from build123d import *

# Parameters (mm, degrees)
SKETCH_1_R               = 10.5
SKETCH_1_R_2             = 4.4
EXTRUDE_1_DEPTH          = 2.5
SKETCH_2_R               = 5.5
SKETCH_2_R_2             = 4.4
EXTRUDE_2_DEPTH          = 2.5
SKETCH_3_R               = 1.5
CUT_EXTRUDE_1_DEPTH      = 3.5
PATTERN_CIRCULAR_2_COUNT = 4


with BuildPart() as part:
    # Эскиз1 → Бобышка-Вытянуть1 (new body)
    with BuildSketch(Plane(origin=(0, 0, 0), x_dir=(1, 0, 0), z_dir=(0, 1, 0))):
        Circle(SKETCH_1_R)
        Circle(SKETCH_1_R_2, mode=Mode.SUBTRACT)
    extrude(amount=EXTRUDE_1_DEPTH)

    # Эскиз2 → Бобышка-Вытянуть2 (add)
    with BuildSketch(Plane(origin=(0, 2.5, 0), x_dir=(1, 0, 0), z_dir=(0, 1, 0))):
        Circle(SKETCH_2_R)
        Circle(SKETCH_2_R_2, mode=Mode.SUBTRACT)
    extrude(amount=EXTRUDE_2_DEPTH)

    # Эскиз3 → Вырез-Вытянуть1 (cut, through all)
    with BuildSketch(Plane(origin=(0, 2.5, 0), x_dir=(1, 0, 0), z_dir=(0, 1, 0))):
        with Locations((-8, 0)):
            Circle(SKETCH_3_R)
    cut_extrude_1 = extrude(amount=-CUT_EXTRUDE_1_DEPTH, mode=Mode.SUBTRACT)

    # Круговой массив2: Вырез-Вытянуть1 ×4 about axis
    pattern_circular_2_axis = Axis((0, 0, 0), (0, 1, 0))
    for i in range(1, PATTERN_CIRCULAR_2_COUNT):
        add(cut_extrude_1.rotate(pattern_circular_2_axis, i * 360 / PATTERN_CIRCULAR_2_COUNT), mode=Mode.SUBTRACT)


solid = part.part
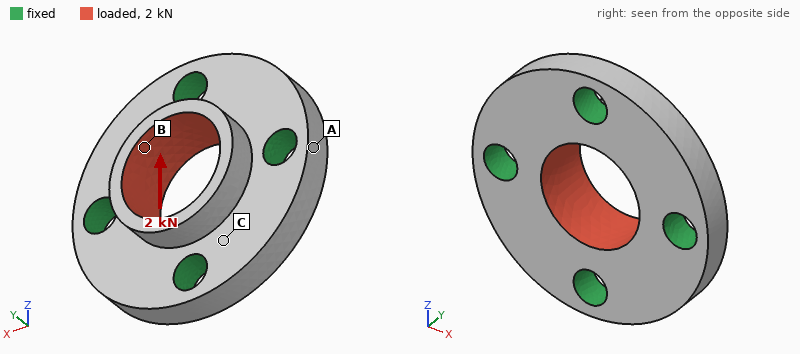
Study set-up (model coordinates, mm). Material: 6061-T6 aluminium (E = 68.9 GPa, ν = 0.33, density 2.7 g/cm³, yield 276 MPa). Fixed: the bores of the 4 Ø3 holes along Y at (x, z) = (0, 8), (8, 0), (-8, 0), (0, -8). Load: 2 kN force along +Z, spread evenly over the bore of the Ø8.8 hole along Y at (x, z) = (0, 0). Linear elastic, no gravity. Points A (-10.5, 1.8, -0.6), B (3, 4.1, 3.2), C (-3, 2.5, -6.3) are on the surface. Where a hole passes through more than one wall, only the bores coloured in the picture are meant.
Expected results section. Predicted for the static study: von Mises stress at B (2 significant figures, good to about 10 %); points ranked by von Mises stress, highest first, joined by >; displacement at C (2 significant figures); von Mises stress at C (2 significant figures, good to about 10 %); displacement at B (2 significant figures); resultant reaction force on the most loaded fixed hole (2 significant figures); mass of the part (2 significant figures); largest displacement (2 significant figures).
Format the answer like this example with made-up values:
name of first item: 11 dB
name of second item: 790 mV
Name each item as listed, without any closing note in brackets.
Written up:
von Mises stress at B: 47 MPa
points ranked by von Mises stress, highest first, joined by >: B > C > A
displacement at C: 1.5 µm
von Mises stress at C: 29 MPa
displacement at B: 6.8 µm
resultant reaction force on the most loaded fixed hole: 550 N
mass of the part: 2.0 g
largest displacement: 9.0 µm
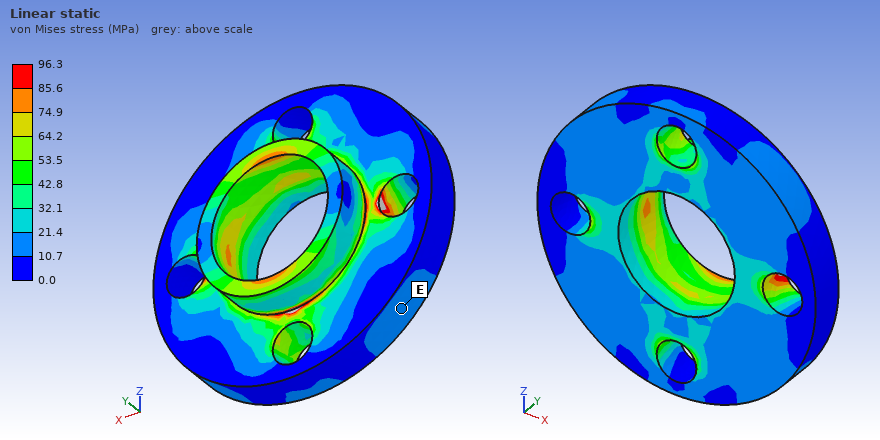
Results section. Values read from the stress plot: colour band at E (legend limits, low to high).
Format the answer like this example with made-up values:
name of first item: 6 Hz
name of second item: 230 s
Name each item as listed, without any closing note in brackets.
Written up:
colour band at E: 10.7 to 21.4 MPa
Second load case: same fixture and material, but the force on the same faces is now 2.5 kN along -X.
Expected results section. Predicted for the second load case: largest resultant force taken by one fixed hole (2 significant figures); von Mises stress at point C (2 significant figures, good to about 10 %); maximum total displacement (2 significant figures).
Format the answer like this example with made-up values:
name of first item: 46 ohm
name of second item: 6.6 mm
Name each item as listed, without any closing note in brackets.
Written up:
largest resultant force taken by one fixed hole: 690 N
von Mises stress at point C: 29 MPa
maximum total displacement: 11 µm
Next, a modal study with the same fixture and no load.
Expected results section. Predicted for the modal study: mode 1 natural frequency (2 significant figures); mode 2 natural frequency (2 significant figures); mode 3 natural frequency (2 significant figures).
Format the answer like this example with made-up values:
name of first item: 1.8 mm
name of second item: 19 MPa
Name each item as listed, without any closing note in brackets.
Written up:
mode 1 natural frequency: 76 kHz
mode 2 natural frequency: 79 kHz
mode 3 natural frequency: 79 kHz
